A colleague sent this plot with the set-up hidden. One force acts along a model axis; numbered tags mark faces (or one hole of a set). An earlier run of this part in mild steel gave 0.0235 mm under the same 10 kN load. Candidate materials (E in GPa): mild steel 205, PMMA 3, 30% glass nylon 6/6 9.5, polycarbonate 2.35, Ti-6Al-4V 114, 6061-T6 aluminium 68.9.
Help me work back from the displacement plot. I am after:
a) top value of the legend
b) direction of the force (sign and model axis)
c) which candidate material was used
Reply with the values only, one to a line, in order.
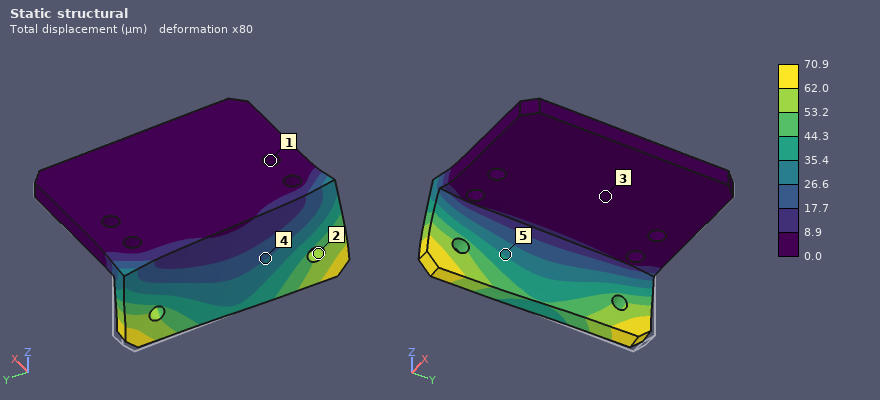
70.9 µm
-Y
6061-T6 aluminium
